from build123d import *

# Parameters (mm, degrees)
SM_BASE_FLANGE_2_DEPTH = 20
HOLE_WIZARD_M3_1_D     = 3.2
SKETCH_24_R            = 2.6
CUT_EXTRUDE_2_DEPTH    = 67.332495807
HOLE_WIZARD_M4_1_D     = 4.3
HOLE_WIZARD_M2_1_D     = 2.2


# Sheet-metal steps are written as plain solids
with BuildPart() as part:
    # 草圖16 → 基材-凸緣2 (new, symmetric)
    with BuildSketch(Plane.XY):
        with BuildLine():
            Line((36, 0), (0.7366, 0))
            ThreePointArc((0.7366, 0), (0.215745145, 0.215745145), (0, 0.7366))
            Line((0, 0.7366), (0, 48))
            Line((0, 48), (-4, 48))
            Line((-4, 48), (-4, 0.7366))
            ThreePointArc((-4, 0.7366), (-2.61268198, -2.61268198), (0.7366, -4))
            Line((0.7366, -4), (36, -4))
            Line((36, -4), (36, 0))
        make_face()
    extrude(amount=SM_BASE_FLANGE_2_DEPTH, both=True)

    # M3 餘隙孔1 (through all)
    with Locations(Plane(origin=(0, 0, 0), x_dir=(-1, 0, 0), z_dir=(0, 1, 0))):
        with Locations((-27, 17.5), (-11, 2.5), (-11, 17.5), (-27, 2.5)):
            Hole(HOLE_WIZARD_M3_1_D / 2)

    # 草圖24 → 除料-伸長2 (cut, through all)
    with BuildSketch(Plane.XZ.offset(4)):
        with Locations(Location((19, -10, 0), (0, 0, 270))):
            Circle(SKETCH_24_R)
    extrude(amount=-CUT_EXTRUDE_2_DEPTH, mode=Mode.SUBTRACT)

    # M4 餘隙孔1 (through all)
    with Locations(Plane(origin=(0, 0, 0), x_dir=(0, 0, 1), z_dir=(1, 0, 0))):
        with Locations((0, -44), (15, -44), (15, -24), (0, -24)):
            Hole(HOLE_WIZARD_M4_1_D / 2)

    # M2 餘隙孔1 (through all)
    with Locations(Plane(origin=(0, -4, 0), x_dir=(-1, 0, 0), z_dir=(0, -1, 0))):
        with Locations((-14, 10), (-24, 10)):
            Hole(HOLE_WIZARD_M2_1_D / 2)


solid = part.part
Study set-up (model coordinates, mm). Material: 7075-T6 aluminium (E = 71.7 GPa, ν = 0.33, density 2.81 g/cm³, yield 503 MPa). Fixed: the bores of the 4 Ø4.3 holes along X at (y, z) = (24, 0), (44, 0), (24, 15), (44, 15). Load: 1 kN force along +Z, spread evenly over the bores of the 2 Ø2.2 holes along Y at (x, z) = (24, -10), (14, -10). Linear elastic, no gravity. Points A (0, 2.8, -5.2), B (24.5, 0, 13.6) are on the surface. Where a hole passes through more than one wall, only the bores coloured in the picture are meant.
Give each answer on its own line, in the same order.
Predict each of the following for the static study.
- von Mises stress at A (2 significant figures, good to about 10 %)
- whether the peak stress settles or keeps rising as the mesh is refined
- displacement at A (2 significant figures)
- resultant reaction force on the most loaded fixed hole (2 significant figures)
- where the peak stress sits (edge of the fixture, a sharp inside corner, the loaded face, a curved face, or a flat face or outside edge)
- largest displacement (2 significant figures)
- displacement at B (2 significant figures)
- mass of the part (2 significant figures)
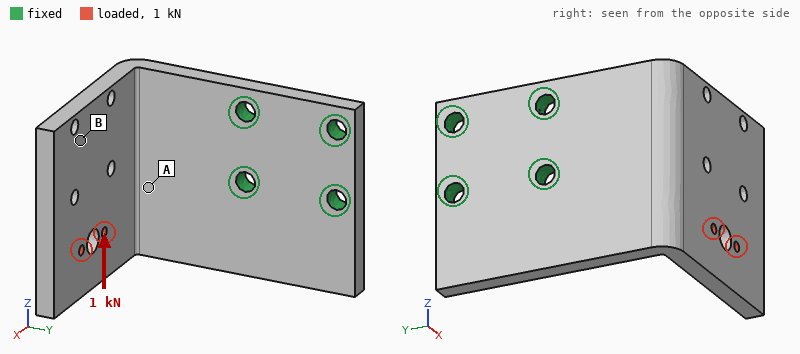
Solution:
110 MPa
keeps rising
0.12 mm
1.6 kN
edge of the fixture
0.73 mm
0.47 mm
38 g
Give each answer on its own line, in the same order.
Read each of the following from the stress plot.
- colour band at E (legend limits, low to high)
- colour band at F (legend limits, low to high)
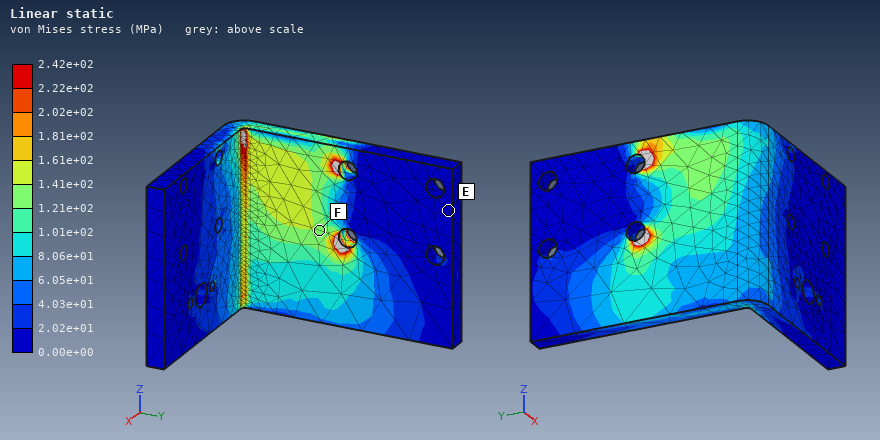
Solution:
0.00e+00 to 2.02e+01 MPa
1.21e+02 to 1.41e+02 MPa
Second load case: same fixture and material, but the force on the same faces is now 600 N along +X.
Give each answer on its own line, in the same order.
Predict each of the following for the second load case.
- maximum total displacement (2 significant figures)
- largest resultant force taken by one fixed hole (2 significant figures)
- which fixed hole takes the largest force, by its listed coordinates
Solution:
0.71 mm
990 N
(24, 0)
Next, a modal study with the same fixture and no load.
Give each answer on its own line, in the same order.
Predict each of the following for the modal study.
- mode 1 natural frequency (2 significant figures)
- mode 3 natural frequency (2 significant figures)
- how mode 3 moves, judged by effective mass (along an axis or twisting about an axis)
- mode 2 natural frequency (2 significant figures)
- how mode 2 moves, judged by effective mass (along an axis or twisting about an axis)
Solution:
1100 Hz
3100 Hz
along X
1800 Hz
along Z
